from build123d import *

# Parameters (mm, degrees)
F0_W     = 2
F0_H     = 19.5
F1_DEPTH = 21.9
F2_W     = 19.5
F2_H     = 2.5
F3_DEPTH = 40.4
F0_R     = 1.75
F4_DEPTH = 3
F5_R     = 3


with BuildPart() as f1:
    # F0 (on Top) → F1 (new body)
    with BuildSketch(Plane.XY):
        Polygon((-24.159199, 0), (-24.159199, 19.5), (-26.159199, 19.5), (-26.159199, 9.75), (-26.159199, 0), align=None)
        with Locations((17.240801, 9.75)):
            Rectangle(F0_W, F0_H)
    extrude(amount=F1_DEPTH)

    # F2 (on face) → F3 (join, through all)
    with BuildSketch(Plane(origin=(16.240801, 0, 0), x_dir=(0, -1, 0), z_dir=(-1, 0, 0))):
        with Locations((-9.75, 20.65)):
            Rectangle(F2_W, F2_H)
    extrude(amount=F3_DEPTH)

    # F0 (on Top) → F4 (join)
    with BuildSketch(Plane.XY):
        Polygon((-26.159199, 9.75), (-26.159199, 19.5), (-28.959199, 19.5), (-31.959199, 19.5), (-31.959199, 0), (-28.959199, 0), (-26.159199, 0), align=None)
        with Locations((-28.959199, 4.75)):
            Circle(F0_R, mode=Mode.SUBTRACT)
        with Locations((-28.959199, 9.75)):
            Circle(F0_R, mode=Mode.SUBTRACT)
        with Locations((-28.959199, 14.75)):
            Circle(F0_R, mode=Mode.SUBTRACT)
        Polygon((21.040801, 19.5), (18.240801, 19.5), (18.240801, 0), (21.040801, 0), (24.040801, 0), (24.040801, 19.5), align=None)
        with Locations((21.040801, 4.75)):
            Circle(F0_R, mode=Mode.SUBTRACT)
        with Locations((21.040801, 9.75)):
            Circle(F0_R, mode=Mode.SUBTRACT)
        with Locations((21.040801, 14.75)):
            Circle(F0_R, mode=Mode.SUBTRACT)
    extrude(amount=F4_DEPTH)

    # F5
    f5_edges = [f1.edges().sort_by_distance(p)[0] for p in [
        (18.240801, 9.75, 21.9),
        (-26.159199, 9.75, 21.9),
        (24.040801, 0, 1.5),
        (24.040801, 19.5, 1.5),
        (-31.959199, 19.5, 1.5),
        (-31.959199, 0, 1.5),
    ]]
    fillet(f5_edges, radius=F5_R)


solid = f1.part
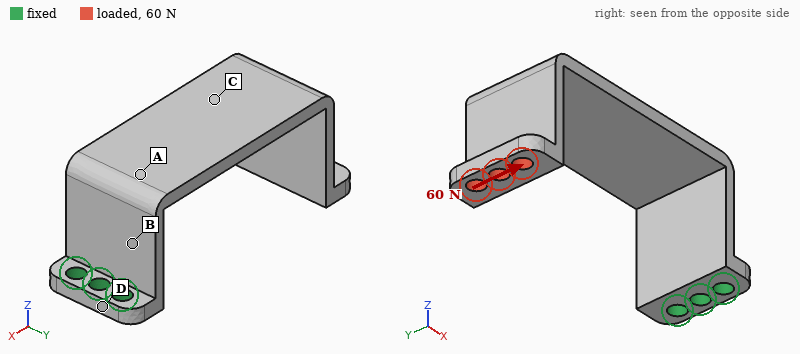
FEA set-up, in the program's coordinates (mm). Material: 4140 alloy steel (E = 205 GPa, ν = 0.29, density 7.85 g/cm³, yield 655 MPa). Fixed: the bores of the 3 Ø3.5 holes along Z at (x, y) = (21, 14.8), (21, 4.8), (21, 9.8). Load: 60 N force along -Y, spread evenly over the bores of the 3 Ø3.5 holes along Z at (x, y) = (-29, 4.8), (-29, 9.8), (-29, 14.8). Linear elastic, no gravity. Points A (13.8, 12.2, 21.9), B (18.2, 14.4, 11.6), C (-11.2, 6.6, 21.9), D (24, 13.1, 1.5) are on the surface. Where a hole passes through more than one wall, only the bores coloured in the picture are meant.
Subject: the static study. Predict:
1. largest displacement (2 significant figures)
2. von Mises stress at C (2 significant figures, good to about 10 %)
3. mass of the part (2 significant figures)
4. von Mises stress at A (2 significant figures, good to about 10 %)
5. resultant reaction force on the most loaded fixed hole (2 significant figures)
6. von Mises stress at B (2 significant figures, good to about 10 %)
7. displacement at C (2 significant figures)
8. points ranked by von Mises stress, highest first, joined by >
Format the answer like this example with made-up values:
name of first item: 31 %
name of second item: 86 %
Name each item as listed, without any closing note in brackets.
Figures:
largest displacement: 0.61 mm
von Mises stress at C: 49 MPa
mass of the part: 32 g
von Mises stress at A: 93 MPa
resultant reaction force on the most loaded fixed hole: 220 N
von Mises stress at B: 160 MPa
displacement at C: 0.25 mm
points ranked by von Mises stress, highest first, joined by >: B > A > C > D
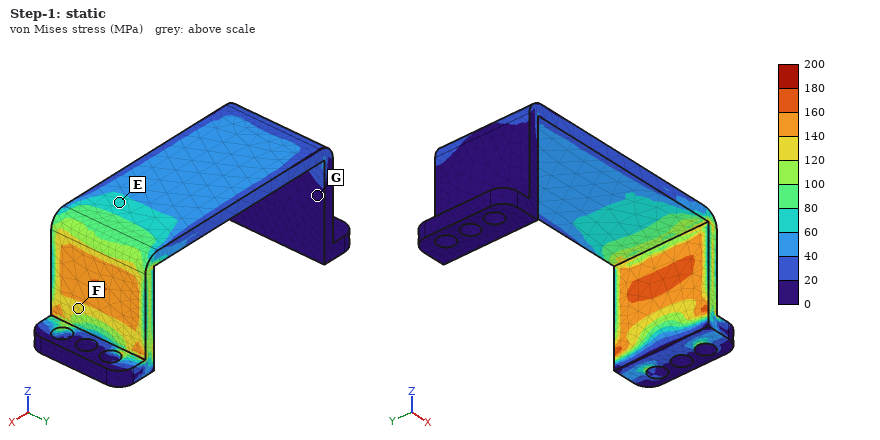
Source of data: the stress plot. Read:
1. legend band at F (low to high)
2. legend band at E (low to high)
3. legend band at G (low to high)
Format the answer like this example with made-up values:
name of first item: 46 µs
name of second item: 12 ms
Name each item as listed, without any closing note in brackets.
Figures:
legend band at F: 120 to 140 MPa
legend band at E: 60 to 80 MPa
legend band at G: 0 to 20 MPa
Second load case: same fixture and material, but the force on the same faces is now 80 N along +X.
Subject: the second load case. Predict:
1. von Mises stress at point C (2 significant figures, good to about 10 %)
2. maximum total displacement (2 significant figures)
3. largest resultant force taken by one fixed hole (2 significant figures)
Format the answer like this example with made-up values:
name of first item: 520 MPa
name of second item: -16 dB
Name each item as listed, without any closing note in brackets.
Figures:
von Mises stress at point C: 71 MPa
maximum total displacement: 0.74 mm
largest resultant force taken by one fixed hole: 36 N
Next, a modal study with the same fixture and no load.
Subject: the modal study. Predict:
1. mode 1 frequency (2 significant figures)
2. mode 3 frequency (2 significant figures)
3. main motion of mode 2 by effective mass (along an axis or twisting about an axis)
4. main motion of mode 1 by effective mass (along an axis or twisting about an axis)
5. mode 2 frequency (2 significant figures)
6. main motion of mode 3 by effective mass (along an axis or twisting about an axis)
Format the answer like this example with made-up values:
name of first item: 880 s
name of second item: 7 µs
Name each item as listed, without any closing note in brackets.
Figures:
mode 1 frequency: 320 Hz
mode 3 frequency: 1200 Hz
main motion of mode 2 by effective mass: along Y
main motion of mode 1 by effective mass: along Z
mode 2 frequency: 540 Hz
main motion of mode 3 by effective mass: along X
